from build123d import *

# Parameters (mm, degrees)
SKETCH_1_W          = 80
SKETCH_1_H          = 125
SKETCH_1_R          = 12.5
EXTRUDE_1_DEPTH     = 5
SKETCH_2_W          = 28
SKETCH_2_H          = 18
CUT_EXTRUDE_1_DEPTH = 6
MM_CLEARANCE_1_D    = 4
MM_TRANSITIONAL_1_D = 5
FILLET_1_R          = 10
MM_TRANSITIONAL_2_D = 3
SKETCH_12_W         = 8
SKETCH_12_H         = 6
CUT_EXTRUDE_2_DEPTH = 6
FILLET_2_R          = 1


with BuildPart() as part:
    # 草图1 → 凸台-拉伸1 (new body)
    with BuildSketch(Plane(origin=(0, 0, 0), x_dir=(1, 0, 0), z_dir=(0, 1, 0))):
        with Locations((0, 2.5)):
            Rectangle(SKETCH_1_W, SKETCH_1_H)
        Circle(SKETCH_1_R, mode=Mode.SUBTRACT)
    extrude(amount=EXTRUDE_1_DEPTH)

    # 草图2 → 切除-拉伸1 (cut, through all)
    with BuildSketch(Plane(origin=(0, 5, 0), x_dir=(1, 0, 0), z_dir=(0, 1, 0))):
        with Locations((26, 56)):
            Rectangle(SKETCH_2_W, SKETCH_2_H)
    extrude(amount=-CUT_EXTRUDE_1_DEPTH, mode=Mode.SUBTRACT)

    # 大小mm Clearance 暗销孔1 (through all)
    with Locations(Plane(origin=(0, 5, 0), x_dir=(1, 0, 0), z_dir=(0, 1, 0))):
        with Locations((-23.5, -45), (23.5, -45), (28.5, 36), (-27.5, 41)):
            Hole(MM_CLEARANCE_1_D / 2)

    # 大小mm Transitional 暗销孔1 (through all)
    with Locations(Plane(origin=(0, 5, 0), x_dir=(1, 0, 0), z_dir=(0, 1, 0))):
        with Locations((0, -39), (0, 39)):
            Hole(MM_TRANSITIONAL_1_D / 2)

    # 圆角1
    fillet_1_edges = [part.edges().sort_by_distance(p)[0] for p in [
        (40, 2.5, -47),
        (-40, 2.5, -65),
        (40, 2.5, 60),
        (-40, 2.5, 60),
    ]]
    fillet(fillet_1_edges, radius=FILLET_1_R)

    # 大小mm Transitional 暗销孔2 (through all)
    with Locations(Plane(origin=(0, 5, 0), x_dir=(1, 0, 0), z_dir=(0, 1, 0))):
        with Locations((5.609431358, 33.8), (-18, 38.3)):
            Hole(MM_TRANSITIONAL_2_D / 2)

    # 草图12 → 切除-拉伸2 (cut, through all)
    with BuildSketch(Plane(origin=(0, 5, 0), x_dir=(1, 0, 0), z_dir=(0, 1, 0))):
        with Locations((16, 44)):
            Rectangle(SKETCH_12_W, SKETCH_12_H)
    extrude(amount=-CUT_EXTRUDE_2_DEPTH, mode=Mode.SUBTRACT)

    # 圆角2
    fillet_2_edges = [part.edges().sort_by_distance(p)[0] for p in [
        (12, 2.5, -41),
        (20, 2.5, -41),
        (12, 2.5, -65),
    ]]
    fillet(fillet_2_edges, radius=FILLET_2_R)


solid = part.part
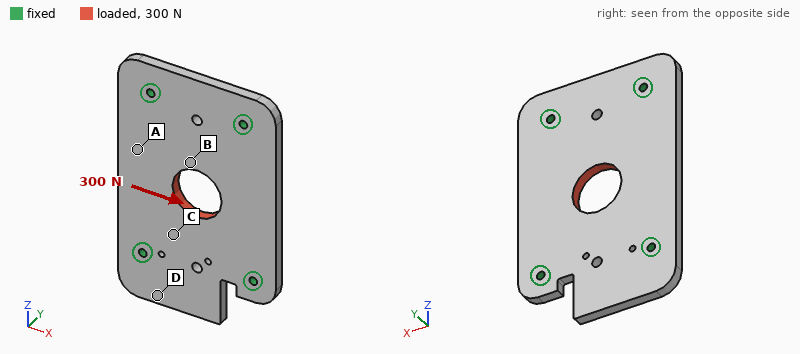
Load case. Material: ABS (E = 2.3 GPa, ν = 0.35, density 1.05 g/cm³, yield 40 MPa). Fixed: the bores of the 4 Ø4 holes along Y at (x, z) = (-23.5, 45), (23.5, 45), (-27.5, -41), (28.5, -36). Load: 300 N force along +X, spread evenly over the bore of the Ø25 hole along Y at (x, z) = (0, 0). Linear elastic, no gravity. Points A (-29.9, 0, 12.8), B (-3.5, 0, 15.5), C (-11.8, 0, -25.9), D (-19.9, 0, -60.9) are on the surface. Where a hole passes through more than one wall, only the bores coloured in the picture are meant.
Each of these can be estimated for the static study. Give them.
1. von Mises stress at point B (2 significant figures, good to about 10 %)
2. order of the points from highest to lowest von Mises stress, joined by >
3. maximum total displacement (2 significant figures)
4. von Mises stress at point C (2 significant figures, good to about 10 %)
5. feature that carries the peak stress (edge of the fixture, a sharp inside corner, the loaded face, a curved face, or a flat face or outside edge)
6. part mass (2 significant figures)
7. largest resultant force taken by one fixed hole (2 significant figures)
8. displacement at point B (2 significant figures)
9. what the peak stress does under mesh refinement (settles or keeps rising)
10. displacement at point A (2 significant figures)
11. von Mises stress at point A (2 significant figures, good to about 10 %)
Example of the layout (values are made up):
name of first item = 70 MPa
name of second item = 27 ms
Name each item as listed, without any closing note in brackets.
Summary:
von Mises stress at point B = 1.1 MPa
order of the points from highest to lowest von Mises stress, joined by > = B > C > A > D
maximum total displacement = 26 µm
von Mises stress at point C = 0.80 MPa
feature that carries the peak stress = edge of the fixture
part mass = 46 g
largest resultant force taken by one fixed hole = 93 N
displacement at point B = 20 µm
what the peak stress does under mesh refinement = keeps rising
displacement at point A = 20 µm
von Mises stress at point A = 0.49 MPa
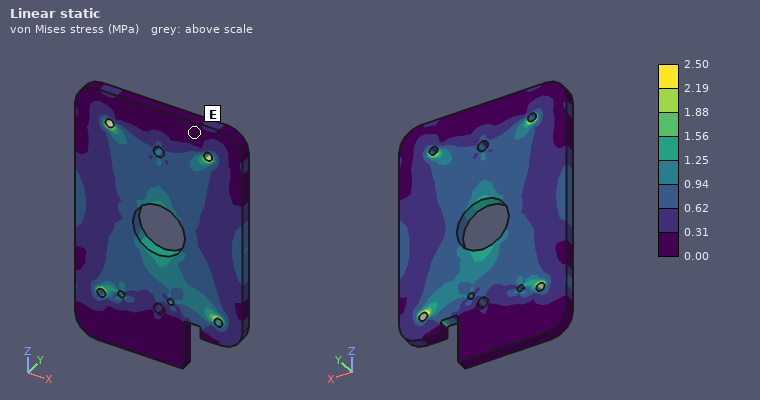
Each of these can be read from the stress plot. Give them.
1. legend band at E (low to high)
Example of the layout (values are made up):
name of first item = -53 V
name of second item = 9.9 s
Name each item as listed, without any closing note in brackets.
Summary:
legend band at E = 0.00 to 0.31 MPa
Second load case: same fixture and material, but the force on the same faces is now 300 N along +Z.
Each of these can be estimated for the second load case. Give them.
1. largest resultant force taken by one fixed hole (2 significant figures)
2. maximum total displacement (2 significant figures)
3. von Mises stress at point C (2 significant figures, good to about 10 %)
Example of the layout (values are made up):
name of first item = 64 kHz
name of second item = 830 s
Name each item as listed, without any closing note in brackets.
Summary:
largest resultant force taken by one fixed hole = 82 N
maximum total displacement = 16 µm
von Mises stress at point C = 0.64 MPa
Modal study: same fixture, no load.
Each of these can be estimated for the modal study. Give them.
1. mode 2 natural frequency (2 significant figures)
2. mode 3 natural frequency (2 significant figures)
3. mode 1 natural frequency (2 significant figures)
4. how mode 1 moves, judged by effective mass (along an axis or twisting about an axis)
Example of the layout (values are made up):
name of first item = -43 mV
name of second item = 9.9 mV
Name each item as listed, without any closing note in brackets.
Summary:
mode 2 natural frequency = 1200 Hz
mode 3 natural frequency = 1200 Hz
mode 1 natural frequency = 910 Hz
how mode 1 moves, judged by effective mass = along Y
